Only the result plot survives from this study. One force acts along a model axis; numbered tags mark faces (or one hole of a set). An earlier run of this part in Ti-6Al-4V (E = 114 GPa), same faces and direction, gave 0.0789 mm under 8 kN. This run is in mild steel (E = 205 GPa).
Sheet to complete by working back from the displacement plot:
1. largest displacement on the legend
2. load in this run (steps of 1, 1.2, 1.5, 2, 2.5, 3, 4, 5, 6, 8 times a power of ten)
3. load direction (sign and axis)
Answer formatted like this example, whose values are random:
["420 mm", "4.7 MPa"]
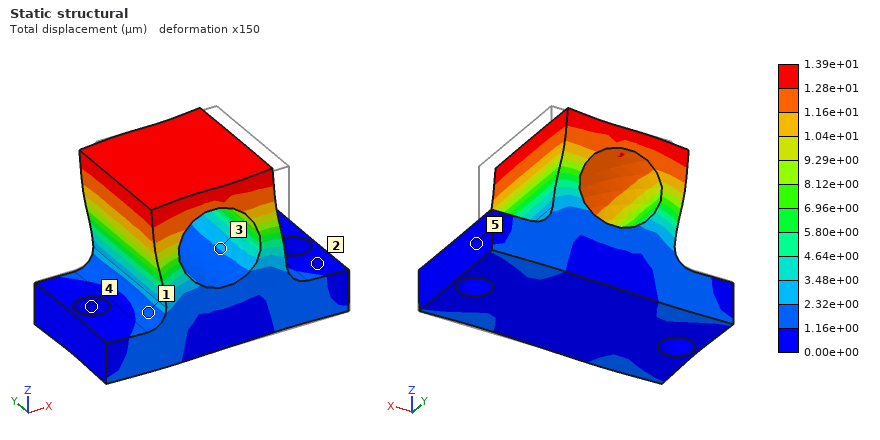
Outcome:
["1.39e+01 µm", "2.5 kN", "-X"]
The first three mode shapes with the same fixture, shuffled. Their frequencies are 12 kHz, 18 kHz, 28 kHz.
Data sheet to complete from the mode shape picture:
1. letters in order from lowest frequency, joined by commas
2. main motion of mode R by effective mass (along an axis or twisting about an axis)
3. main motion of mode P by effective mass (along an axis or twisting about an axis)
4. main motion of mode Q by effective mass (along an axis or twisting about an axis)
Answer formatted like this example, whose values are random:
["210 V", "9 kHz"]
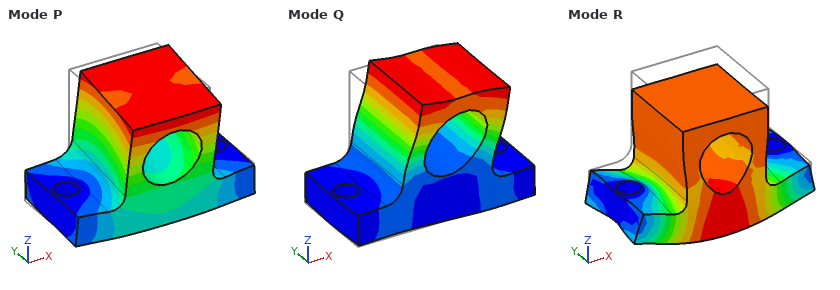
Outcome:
["P, Q, R", "along Z", "along Y", "along X"]
